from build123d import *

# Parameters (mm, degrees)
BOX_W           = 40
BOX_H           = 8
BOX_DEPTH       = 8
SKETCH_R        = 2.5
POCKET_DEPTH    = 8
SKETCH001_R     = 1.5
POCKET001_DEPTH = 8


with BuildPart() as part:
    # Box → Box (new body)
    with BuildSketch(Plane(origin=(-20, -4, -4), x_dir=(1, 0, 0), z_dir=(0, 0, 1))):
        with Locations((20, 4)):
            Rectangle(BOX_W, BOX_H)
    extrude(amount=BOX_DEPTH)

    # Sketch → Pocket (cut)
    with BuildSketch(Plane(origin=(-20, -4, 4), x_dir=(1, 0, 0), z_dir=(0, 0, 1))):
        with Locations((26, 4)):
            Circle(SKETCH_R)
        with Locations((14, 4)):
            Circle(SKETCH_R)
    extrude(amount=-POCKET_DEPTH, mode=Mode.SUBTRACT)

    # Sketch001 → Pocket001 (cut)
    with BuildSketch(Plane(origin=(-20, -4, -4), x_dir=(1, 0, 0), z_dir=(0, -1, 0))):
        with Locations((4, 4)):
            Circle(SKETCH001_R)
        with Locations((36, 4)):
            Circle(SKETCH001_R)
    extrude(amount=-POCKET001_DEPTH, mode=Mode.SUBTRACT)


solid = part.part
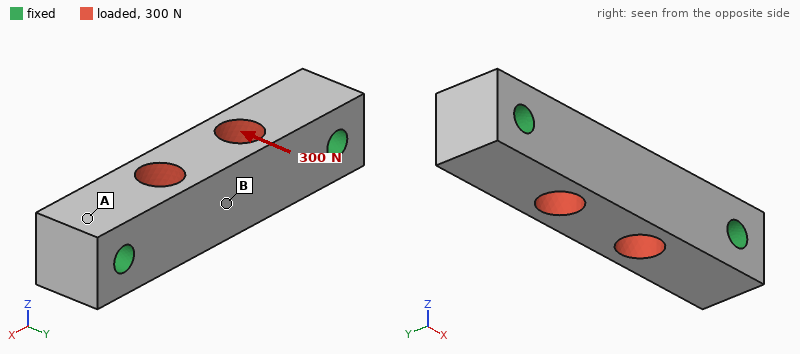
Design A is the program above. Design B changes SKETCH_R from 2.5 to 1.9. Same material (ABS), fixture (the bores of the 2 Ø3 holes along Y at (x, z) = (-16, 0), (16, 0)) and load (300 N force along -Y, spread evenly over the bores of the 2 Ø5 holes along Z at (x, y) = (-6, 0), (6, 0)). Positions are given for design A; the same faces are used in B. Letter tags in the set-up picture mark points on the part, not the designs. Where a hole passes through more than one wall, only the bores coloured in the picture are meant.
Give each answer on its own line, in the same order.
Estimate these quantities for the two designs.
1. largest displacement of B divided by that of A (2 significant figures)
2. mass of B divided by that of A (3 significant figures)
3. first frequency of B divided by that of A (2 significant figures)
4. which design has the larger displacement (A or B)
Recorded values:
0.73
1.06
1.0
A
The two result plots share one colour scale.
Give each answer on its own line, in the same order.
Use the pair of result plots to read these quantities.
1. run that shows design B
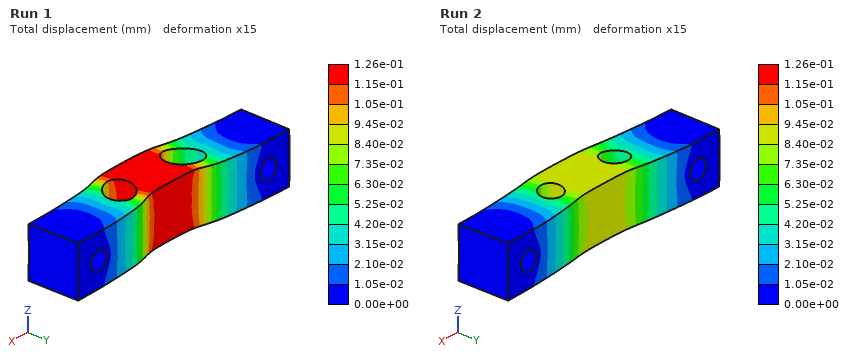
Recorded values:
Run 2
